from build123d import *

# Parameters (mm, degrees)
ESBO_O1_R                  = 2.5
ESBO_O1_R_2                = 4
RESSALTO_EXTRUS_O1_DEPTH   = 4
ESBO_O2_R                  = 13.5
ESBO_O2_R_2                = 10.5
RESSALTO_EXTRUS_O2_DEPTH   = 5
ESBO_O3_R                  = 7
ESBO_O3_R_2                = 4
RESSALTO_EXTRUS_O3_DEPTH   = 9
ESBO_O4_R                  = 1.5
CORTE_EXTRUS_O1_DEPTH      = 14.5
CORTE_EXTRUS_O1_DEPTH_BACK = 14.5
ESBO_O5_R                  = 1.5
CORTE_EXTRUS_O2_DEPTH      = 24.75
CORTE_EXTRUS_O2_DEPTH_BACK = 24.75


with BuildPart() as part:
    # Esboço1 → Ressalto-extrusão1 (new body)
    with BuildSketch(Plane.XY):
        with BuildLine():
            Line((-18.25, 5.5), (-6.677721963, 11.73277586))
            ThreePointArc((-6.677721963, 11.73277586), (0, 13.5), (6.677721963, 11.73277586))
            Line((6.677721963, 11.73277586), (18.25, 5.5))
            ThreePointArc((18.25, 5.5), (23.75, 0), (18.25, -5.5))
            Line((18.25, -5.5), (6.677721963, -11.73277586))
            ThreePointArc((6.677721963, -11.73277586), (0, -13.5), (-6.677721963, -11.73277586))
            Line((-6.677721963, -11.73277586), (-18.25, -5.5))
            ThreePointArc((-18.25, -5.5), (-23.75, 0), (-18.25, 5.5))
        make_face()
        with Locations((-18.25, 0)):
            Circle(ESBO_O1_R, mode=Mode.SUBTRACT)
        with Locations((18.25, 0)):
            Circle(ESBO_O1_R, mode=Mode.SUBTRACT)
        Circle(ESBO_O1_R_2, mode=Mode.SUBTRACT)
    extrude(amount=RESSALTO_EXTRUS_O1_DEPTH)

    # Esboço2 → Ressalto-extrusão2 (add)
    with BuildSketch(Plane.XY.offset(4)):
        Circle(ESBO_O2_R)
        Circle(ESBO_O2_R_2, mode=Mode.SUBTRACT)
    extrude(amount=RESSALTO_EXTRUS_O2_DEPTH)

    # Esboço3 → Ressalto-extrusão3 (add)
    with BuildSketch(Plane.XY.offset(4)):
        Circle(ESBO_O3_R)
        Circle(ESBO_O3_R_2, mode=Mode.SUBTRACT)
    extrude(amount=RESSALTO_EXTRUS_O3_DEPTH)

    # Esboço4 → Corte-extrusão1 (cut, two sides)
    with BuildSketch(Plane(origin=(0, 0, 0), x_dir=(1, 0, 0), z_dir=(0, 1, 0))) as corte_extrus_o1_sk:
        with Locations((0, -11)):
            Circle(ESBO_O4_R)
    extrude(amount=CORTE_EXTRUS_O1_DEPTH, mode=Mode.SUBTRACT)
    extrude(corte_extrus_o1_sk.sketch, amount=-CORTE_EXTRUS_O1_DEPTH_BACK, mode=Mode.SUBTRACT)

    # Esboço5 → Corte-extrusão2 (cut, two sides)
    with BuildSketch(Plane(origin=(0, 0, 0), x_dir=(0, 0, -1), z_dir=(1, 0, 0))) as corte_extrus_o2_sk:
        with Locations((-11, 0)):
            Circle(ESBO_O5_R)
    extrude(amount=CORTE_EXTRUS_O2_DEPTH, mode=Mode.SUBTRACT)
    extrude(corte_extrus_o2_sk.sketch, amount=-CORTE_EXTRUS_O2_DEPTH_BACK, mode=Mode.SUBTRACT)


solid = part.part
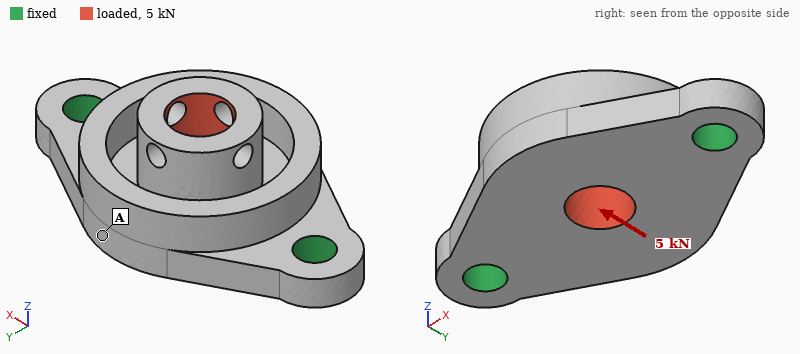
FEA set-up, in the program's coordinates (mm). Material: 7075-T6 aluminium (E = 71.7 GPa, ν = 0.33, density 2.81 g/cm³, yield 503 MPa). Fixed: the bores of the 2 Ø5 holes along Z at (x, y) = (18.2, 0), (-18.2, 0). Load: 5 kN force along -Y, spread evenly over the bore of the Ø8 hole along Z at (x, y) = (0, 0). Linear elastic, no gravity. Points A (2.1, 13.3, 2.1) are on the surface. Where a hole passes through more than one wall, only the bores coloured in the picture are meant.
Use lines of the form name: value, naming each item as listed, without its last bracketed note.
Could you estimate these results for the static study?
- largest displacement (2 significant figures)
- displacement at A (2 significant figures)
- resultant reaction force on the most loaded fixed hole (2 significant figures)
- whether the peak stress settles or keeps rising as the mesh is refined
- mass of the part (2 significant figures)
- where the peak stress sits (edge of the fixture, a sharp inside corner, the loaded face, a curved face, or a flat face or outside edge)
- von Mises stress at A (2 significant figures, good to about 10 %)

largest displacement: 0.15 mm
displacement at A: 0.100 mm
resultant reaction force on the most loaded fixed hole: 2.5 kN
whether the peak stress settles or keeps rising as the mesh is refined: keeps rising
mass of the part: 14 g
where the peak stress sits: edge of the fixture
von Mises stress at A: 54 MPa
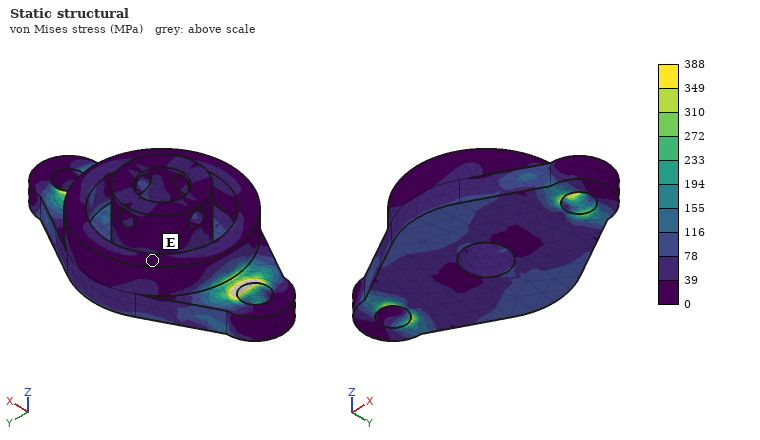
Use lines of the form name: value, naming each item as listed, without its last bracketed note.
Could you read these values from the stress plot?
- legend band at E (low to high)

legend band at E: 0 to 39 MPa
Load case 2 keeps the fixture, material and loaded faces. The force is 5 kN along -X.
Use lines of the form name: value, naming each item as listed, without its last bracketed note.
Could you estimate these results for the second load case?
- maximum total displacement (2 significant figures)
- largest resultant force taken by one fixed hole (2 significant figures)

maximum total displacement: 45 µm
largest resultant force taken by one fixed hole: 2.6 kN
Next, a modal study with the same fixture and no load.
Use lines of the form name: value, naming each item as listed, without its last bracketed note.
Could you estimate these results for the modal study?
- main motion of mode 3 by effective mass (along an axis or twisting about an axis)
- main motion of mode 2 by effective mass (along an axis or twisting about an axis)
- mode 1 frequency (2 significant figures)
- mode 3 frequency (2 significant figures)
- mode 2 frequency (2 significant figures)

main motion of mode 3 by effective mass: along Y
main motion of mode 2 by effective mass: along Z
mode 1 frequency: 9500 Hz
mode 3 frequency: 26 kHz
mode 2 frequency: 13 kHz
